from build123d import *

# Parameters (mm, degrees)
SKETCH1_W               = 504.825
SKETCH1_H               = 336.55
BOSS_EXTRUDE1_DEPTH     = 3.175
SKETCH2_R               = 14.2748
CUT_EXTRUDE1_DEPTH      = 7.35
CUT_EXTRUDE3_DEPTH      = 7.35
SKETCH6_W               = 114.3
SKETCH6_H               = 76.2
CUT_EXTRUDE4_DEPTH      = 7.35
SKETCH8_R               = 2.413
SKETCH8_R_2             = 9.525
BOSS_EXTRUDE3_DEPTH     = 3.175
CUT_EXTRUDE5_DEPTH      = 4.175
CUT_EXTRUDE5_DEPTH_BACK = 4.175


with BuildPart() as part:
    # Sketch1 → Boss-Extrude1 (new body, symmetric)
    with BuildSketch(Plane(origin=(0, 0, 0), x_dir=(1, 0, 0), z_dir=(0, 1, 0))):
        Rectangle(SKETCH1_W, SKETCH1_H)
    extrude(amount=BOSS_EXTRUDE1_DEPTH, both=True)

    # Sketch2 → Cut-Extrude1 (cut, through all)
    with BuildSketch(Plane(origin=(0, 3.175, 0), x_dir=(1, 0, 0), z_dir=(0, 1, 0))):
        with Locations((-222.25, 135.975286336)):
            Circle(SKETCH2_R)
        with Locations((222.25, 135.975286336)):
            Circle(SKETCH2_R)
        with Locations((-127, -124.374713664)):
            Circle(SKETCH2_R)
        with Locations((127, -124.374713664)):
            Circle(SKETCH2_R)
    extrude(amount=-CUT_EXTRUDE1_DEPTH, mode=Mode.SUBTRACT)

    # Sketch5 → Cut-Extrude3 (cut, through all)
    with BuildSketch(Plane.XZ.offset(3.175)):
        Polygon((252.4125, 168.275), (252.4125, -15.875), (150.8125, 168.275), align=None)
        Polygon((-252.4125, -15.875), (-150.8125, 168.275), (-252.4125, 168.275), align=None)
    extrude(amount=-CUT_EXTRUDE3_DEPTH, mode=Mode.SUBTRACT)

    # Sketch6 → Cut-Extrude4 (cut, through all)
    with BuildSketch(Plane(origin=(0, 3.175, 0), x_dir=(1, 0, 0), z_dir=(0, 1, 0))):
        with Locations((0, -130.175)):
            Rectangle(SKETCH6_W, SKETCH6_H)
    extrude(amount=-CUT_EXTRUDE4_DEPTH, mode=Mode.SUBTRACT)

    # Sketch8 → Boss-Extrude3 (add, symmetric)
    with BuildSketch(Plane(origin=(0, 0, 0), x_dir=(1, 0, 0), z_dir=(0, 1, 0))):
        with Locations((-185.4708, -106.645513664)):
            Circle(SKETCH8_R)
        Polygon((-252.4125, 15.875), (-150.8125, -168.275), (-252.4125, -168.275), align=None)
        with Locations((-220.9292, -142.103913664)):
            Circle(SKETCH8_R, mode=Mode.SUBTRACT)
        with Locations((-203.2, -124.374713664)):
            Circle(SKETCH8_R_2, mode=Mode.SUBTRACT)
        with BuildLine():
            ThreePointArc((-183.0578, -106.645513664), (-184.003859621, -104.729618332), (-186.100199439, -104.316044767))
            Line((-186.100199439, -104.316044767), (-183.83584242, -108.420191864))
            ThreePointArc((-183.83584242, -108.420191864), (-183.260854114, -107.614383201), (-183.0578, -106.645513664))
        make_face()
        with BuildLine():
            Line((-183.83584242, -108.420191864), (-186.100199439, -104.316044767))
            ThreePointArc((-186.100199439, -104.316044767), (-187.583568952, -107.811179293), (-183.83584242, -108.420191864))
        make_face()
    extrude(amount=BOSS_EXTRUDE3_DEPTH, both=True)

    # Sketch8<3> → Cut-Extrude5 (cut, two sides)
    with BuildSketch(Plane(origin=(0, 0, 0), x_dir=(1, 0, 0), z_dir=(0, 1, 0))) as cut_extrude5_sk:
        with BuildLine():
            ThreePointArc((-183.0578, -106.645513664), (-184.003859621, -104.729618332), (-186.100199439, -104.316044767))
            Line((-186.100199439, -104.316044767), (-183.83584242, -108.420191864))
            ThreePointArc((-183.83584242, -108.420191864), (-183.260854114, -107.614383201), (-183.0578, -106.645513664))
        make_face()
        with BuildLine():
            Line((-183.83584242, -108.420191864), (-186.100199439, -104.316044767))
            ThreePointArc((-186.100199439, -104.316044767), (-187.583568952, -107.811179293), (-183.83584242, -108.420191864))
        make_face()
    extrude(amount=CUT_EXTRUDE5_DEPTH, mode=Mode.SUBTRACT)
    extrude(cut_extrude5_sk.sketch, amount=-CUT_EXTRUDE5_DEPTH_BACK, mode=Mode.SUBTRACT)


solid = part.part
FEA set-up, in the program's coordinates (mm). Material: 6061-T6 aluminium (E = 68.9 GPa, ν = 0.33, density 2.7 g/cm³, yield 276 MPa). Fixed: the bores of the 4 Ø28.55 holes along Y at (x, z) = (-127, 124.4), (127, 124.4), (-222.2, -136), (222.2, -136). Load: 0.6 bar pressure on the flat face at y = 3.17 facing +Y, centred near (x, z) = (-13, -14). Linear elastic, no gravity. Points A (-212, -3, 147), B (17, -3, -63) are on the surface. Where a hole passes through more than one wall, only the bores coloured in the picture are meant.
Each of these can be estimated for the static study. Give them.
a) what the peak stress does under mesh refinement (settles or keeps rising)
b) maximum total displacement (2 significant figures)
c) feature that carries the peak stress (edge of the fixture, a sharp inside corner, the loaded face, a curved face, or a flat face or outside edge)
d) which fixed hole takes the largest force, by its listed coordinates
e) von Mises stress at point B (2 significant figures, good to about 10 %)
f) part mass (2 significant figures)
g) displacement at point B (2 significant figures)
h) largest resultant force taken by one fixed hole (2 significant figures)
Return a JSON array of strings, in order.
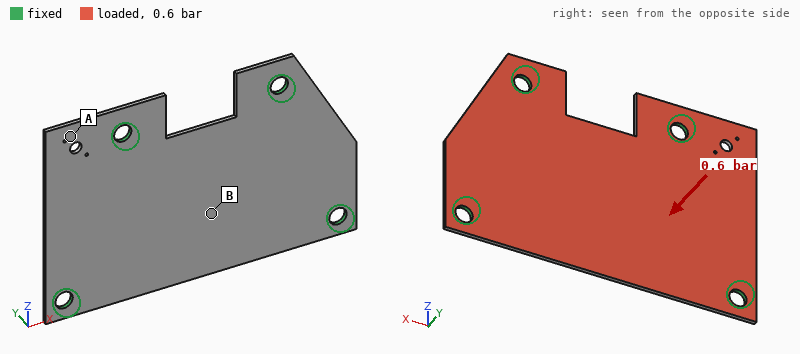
["keeps rising", "3.7 mm", "edge of the fixture", "(-127, 124.4)", "45 MPa", "2.6 kg", "2.8 mm", "2.5 kN"]
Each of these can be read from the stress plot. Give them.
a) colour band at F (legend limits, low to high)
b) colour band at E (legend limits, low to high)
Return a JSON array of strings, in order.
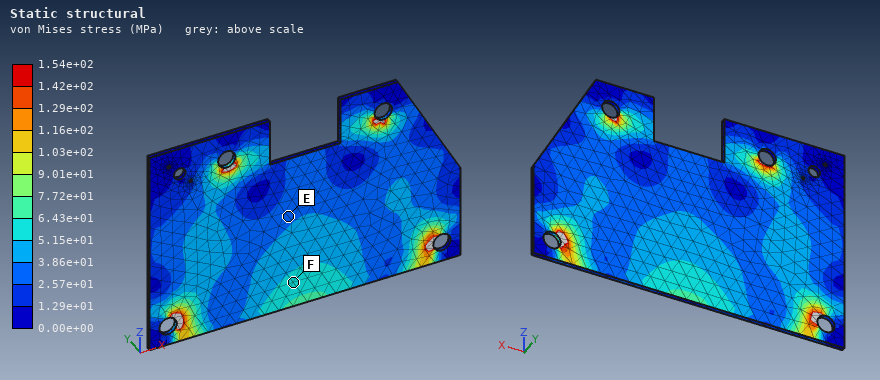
["5.15e+01 to 6.43e+01 MPa", "2.57e+01 to 3.86e+01 MPa"]
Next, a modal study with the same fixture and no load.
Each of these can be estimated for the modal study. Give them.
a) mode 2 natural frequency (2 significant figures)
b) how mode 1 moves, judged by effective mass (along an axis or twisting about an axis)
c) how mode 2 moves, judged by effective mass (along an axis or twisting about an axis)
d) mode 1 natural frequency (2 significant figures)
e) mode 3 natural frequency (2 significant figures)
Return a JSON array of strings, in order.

["380 Hz", "along Y", "along Y", "200 Hz", "430 Hz"]
